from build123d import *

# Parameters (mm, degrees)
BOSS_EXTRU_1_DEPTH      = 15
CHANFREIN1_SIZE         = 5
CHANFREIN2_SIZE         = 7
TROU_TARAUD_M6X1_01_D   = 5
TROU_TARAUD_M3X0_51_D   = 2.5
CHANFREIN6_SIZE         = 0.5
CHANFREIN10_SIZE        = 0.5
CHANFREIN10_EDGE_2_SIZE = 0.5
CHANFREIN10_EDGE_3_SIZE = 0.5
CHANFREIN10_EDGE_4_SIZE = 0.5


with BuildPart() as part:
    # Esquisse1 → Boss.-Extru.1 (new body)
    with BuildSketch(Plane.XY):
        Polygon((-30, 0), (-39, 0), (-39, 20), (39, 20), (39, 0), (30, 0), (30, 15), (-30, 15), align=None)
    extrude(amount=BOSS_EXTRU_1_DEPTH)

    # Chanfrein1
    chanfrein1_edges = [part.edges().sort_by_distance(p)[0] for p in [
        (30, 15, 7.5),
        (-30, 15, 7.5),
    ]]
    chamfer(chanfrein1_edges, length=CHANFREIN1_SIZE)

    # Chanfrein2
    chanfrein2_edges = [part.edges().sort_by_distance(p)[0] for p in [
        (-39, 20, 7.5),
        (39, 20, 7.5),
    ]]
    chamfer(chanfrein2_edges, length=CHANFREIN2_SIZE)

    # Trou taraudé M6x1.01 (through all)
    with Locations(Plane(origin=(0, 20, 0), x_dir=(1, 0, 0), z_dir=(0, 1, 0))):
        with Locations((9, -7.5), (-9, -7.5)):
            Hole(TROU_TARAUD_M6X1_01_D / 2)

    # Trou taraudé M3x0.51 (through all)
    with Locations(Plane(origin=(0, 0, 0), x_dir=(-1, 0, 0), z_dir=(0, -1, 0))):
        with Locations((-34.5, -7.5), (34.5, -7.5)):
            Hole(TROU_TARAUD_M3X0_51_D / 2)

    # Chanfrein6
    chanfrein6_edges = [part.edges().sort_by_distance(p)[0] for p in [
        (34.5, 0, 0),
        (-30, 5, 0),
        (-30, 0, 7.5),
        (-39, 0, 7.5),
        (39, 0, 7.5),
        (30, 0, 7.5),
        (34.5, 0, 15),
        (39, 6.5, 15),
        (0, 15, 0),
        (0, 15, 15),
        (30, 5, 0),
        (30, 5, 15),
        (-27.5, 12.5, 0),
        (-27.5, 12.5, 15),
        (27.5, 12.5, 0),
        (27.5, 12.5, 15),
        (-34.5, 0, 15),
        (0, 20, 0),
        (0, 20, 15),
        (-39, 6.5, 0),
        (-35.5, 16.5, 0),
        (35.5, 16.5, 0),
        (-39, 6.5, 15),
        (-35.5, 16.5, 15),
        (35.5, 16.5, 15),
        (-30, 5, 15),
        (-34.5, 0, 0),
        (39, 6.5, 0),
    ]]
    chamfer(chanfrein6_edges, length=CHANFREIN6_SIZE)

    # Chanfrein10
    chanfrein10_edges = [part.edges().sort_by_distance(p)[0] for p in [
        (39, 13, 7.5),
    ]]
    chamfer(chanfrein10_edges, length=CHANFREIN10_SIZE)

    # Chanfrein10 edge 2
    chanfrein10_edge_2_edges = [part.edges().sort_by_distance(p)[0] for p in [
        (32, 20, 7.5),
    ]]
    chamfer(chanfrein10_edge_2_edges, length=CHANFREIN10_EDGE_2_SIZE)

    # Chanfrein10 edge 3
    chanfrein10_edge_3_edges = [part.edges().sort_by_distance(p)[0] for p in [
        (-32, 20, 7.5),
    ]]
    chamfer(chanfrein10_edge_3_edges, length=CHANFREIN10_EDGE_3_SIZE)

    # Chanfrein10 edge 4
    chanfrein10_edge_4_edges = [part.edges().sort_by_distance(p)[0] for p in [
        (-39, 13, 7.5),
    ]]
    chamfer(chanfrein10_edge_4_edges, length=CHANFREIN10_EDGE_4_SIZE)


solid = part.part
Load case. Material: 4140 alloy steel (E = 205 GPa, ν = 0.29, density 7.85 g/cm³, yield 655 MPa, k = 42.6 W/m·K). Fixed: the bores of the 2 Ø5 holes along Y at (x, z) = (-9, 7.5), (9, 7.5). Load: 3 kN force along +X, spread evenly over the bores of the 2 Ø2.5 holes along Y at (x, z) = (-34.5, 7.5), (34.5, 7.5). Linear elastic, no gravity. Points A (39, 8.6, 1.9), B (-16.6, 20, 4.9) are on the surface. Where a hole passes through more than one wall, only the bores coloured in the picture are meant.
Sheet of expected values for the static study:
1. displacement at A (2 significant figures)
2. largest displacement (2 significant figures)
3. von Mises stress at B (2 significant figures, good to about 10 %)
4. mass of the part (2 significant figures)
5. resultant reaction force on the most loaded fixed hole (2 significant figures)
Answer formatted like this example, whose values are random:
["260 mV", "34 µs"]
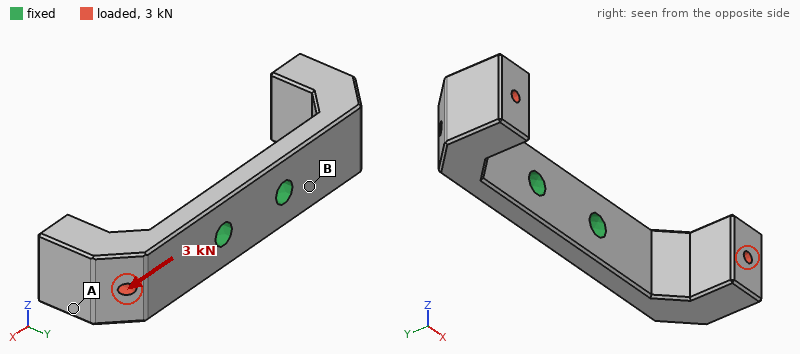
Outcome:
["0.16 mm", "0.20 mm", "180 MPa", "71 g", "1.5 kN"]
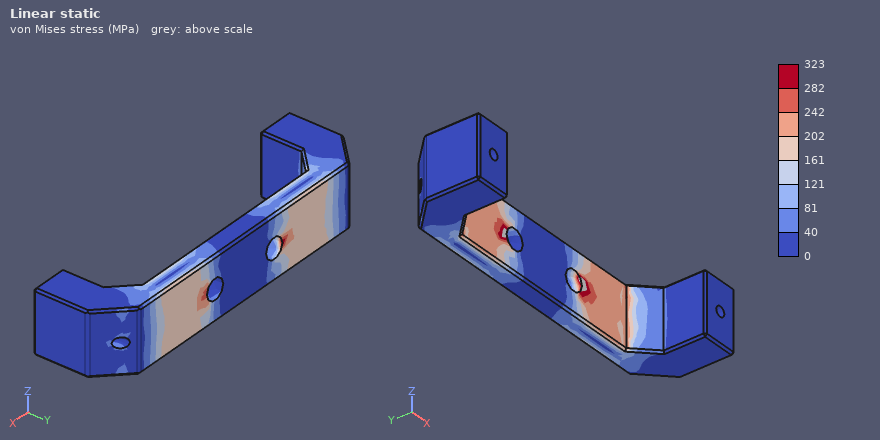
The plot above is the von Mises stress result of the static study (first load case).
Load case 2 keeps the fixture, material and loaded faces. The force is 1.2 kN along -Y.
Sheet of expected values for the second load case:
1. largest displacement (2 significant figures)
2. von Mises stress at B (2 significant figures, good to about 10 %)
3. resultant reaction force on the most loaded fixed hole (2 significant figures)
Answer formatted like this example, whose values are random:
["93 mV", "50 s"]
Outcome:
["0.15 mm", "160 MPa", "600 N"]
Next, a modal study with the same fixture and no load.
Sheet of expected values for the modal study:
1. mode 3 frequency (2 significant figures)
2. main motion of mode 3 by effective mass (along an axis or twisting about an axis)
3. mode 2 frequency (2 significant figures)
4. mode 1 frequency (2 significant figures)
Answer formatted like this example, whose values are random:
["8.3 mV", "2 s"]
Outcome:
["4400 Hz", "twisting about Y", "2600 Hz", "2600 Hz"]
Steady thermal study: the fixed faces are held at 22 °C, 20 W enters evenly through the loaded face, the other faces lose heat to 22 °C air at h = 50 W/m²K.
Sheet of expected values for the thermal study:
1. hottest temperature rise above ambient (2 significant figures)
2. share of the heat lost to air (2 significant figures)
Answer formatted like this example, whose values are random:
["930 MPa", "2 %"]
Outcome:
["57 K", "33 %"]
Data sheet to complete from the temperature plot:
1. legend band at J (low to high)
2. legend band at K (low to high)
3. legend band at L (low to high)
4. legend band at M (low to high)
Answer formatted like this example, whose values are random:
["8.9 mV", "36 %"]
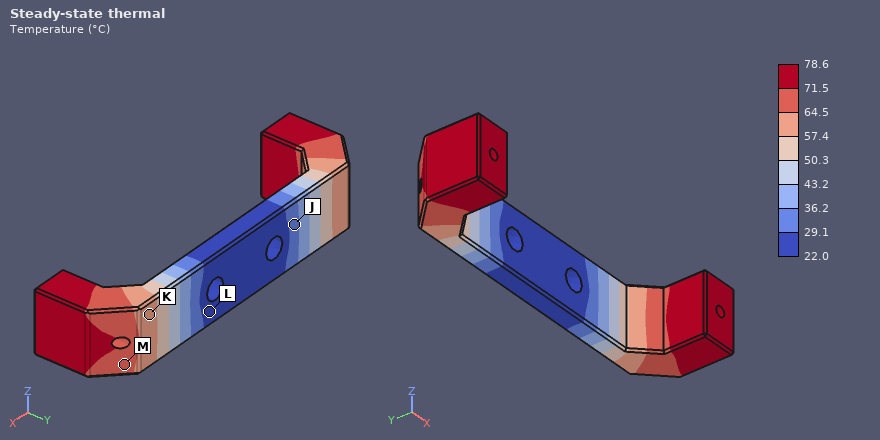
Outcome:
["29.1 to 36.2 °C", "57.4 to 64.5 °C", "22.0 to 29.1 °C", "64.5 to 71.5 °C"]
